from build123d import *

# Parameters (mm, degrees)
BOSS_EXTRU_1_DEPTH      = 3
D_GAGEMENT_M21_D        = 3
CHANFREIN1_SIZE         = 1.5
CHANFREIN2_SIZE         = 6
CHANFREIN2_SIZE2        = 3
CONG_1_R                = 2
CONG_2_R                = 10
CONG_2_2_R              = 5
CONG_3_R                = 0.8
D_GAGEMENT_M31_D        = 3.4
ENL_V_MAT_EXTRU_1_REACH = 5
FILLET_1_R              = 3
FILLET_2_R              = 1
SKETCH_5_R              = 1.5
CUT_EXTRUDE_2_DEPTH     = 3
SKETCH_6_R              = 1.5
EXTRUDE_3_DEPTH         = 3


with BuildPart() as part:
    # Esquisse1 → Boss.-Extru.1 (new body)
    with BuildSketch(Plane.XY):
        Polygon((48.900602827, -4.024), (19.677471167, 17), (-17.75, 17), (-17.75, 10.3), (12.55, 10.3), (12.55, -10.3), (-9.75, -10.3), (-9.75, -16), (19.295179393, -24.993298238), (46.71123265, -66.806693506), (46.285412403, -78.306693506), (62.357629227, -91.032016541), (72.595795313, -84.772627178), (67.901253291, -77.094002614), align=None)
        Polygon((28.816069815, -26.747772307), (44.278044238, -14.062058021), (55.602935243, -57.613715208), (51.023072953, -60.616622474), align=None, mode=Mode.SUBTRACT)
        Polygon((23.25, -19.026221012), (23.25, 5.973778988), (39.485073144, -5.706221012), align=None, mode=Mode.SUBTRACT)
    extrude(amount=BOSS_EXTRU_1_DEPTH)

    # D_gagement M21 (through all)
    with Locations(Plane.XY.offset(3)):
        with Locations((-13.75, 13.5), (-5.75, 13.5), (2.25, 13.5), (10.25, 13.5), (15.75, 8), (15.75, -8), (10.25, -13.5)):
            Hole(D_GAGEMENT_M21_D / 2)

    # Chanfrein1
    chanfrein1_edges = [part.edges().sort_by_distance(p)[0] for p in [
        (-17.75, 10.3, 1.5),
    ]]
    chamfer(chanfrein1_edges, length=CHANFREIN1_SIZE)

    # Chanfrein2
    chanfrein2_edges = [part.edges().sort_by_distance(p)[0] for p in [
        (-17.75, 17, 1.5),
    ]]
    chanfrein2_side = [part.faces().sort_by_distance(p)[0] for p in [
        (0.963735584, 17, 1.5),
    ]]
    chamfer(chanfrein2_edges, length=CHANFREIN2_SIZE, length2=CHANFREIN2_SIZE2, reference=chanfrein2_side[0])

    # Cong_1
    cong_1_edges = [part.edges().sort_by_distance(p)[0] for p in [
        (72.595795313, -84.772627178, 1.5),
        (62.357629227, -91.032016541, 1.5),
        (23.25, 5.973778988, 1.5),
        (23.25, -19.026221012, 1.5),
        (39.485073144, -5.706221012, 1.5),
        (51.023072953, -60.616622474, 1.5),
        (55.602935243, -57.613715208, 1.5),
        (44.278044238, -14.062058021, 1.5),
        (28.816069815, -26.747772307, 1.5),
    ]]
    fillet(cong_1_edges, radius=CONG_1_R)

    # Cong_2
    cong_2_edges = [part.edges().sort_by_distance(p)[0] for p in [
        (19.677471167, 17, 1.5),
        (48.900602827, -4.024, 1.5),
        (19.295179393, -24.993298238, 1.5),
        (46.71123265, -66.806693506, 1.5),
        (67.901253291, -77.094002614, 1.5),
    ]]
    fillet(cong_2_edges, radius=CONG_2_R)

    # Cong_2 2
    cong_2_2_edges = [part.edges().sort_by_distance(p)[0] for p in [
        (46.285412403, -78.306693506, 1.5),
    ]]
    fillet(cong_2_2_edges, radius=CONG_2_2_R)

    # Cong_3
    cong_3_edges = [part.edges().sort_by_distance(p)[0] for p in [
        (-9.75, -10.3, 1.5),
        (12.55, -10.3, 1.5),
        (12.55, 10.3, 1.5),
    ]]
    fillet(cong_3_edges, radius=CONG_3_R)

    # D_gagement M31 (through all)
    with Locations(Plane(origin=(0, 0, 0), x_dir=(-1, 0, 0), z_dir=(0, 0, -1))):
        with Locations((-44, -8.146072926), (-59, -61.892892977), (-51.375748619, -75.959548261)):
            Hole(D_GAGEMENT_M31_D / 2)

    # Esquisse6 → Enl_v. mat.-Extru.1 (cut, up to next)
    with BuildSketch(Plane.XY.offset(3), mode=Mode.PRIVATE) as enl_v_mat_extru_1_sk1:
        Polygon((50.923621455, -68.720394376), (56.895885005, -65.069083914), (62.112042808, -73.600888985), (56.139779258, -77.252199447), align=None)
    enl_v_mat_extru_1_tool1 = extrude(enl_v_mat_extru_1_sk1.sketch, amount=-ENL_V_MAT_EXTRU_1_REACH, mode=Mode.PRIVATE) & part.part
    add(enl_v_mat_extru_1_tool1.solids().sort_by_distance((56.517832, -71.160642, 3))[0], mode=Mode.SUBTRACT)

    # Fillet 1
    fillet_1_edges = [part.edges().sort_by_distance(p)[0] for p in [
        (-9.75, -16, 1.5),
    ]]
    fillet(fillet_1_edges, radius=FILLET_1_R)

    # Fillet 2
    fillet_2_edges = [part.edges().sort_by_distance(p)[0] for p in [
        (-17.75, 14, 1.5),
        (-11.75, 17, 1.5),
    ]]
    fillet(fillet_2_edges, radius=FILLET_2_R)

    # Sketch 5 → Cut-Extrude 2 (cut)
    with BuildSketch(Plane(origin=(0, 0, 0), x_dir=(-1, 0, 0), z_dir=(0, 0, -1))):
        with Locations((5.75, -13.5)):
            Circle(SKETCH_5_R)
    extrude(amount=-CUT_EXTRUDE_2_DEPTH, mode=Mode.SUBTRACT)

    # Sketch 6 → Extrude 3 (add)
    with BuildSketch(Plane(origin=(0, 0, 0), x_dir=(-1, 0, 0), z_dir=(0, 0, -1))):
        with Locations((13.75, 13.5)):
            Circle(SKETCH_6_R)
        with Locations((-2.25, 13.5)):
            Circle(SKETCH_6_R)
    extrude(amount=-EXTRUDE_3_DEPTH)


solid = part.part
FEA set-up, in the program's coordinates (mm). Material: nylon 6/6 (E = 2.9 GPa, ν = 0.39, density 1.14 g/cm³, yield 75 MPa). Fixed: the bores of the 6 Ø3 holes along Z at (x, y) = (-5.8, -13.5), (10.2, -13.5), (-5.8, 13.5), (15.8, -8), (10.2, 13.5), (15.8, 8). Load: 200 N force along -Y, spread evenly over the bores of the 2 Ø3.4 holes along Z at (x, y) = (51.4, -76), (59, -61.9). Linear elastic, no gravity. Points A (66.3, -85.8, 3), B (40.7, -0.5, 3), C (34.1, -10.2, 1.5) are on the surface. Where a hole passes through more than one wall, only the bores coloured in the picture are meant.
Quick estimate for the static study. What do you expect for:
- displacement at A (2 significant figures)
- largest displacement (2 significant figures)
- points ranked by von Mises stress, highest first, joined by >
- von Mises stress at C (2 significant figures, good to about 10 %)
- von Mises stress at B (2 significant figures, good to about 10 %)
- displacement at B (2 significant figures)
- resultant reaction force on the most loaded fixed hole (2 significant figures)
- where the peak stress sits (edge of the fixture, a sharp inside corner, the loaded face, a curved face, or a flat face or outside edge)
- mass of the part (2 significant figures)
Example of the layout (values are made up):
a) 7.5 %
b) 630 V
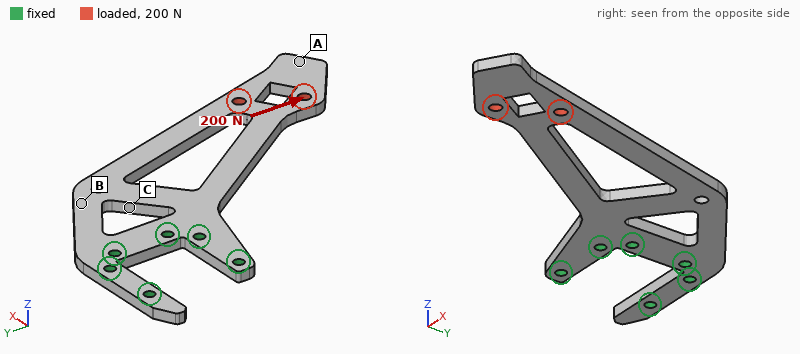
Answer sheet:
a) 1.5 mm
b) 1.5 mm
c) B > C > A
d) 5.8 MPa
e) 10 MPa
f) 0.23 mm
g) 200 N
h) a curved face
i) 8.1 g
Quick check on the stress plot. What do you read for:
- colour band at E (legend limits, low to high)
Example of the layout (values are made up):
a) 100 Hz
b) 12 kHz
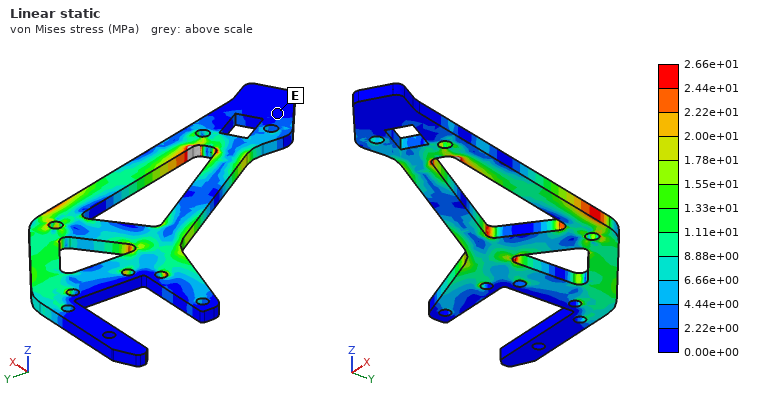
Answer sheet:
a) 0.00e+00 to 2.22e+00 MPa
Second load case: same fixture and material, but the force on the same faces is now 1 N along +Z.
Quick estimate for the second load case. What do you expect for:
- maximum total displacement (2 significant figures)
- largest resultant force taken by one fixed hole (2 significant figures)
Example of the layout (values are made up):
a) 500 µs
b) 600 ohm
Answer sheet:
a) 1.7 mm
b) 1.5 N
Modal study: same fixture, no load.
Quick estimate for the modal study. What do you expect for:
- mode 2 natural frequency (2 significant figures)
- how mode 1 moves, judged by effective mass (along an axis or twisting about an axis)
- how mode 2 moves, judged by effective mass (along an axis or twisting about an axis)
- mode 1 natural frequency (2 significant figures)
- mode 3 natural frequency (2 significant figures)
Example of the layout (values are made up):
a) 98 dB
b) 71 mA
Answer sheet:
a) 430 Hz
b) along Z
c) along Z
d) 93 Hz
e) 690 Hz
